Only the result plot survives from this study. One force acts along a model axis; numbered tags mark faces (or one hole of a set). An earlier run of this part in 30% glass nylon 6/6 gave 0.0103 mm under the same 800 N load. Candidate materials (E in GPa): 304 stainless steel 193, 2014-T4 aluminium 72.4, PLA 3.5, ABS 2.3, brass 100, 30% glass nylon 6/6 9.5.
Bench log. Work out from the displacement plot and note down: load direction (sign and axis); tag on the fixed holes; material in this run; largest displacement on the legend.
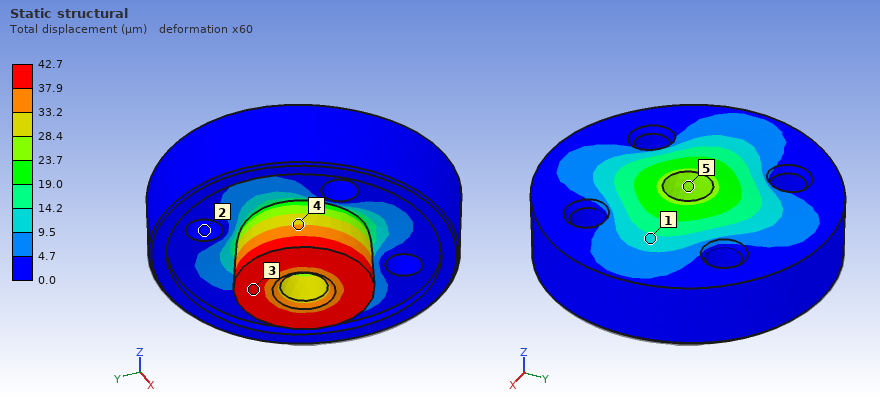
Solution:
+Z
2
ABS
42.7 µm
